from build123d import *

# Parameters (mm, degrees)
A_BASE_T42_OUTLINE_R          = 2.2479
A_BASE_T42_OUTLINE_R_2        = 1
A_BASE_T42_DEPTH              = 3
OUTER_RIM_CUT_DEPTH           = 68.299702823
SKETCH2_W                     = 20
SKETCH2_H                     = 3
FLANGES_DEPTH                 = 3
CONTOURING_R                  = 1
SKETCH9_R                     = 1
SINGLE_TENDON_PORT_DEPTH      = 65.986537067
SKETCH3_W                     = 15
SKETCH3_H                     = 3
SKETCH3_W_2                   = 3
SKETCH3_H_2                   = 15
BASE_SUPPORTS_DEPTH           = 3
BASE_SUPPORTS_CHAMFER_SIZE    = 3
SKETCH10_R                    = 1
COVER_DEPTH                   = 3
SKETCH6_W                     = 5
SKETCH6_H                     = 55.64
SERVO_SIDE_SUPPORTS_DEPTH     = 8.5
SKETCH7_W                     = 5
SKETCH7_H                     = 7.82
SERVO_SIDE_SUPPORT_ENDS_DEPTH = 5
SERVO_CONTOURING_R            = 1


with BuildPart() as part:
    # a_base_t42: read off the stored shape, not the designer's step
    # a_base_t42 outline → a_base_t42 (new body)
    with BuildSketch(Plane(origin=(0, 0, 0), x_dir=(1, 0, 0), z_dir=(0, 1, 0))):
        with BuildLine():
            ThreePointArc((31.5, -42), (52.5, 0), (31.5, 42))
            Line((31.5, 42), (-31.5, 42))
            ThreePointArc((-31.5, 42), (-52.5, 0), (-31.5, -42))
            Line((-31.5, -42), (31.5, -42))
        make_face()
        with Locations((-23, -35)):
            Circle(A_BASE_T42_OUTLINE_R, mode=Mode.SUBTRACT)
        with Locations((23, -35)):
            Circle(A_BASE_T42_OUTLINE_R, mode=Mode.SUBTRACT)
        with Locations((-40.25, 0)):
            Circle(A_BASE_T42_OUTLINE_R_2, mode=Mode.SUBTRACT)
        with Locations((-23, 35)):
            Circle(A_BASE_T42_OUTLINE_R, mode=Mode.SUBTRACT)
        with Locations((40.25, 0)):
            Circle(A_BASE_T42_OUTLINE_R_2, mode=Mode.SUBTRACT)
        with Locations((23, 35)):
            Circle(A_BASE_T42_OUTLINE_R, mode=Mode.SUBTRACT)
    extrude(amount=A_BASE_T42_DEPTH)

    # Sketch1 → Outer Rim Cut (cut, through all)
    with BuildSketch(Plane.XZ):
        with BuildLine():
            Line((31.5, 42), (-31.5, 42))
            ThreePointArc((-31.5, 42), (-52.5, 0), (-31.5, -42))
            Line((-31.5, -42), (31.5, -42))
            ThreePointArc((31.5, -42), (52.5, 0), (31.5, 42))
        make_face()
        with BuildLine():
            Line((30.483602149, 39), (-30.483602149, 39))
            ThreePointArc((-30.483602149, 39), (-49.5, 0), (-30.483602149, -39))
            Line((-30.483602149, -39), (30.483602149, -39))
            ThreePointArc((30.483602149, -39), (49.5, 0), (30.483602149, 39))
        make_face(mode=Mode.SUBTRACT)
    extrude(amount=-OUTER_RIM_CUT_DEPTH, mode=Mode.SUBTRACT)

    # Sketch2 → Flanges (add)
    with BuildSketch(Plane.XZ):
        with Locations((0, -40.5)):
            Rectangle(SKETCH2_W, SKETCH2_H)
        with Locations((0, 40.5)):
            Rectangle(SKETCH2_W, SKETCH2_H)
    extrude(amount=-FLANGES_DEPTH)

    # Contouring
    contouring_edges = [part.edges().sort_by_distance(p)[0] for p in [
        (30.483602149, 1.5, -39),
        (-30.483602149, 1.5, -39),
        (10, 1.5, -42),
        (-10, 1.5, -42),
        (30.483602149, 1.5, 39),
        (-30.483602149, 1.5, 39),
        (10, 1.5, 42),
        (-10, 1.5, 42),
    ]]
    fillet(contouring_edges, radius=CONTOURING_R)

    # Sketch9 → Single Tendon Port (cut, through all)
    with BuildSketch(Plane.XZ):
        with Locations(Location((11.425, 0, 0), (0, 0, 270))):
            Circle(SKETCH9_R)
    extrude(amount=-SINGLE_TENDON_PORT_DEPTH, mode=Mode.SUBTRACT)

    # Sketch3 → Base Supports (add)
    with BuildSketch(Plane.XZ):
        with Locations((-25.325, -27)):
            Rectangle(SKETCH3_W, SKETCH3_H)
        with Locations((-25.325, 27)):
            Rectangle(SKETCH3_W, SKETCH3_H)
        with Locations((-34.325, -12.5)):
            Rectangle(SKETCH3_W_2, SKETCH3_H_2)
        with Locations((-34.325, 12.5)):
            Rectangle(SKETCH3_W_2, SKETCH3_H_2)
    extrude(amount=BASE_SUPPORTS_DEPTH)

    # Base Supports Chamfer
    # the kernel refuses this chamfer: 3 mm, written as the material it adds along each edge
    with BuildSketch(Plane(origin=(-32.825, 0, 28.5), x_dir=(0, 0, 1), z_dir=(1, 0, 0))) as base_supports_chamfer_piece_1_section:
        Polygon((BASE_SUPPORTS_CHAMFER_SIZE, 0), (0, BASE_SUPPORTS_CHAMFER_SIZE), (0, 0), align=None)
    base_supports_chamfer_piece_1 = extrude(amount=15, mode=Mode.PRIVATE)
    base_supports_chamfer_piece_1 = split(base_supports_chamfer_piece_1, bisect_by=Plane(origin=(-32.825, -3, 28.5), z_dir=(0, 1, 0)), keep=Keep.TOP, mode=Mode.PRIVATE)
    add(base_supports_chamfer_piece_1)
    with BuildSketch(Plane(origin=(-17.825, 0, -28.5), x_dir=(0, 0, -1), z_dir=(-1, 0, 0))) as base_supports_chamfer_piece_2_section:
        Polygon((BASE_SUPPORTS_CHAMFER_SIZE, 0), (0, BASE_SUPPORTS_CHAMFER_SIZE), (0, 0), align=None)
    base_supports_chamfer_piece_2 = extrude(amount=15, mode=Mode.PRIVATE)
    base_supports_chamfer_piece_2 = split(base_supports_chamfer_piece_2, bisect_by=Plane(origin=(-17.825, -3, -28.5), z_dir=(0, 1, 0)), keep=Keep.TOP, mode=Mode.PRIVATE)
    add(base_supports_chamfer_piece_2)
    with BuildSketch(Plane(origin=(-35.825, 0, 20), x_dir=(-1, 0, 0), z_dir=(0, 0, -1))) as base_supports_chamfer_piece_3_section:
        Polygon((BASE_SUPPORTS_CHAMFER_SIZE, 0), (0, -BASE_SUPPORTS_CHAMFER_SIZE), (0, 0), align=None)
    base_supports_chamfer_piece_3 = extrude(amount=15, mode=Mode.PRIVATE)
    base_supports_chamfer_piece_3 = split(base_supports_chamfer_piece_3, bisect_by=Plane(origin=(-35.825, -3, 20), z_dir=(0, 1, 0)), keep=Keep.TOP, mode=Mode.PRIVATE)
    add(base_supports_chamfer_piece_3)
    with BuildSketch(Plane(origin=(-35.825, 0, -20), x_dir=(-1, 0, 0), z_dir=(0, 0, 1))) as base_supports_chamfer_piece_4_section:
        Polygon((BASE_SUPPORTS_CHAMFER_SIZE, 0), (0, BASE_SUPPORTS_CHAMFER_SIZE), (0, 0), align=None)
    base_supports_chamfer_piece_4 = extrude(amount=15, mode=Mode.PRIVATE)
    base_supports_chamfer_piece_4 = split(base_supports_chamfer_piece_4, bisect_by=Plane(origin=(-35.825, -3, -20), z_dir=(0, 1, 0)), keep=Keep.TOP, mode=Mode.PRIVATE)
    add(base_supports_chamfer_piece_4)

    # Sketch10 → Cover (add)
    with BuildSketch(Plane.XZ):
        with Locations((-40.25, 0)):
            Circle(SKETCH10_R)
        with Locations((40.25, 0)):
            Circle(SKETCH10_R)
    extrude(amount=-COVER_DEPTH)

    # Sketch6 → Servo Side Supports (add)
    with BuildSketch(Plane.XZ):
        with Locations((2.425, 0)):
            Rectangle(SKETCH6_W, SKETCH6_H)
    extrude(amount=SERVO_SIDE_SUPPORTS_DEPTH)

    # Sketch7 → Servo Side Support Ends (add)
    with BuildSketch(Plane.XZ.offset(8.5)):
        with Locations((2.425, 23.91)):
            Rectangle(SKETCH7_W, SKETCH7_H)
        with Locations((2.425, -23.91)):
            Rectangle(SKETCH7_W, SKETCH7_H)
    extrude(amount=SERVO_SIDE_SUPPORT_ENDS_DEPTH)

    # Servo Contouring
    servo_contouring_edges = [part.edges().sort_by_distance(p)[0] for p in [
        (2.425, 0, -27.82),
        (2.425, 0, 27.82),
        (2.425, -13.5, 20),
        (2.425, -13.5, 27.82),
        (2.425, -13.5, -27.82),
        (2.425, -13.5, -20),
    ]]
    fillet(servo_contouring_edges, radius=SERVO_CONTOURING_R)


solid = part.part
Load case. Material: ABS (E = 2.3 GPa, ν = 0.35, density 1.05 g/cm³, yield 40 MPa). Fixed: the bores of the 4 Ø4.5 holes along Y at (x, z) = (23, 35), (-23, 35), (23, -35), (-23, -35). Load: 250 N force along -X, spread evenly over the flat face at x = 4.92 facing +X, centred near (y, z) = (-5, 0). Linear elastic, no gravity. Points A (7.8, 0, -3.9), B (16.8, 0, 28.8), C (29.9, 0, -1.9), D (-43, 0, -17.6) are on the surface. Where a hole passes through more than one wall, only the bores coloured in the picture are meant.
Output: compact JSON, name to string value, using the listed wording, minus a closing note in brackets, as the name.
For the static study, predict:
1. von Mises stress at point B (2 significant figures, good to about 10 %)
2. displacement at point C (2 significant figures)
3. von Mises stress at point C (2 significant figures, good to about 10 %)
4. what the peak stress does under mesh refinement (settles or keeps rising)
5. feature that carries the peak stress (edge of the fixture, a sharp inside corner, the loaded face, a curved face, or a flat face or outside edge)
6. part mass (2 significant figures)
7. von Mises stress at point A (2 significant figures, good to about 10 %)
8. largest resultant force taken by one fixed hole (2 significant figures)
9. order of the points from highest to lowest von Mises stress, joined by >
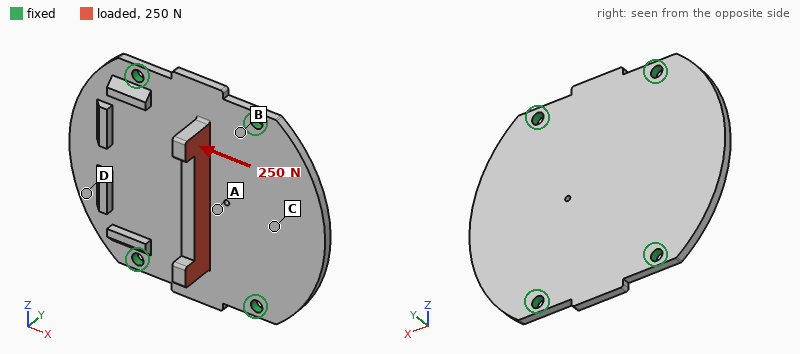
{"von Mises stress at point B": "2.4 MPa", "displacement at point C": "0.15 mm", "von Mises stress at point C": "1.3 MPa", "what the peak stress does under mesh refinement": "keeps rising", "feature that carries the peak stress": "a sharp inside corner", "part mass": "25 g", "von Mises stress at point A": "4.9 MPa", "largest resultant force taken by one fixed hole": "70 N", "order of the points from highest to lowest von Mises stress, joined by >": "A > B > C > D"}
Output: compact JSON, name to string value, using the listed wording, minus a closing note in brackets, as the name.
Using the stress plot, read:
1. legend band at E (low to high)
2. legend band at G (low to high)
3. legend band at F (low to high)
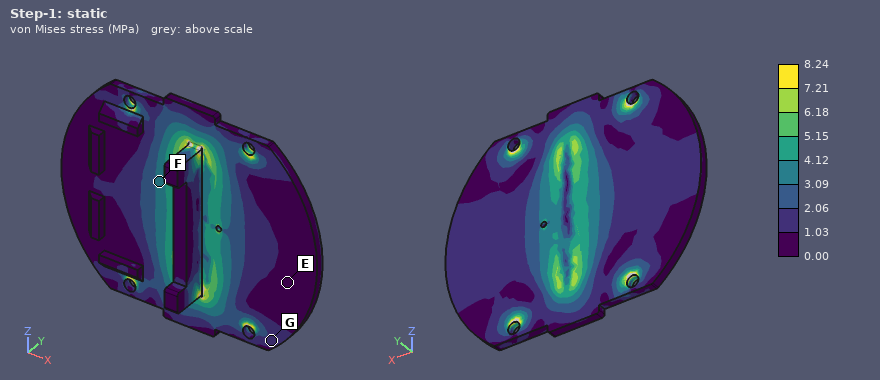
{"legend band at E": "0.00 to 1.03 MPa", "legend band at G": "1.03 to 2.06 MPa", "legend band at F": "3.09 to 4.12 MPa"}
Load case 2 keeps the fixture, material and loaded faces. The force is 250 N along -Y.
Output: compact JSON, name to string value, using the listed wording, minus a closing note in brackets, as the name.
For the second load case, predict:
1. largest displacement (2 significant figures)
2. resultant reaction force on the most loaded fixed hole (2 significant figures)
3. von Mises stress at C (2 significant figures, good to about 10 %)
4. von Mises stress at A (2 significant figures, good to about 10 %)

{"largest displacement": "0.67 mm", "resultant reaction force on the most loaded fixed hole": "82 N", "von Mises stress at C": "3.1 MPa", "von Mises stress at A": "8.2 MPa"}
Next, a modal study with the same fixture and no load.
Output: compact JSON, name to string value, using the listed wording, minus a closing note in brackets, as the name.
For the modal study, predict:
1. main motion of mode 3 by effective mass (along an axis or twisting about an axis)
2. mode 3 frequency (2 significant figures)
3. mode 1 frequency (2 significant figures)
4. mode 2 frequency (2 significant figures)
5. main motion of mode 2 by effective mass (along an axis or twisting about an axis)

{"main motion of mode 3 by effective mass": "along Y", "mode 3 frequency": "1100 Hz", "mode 1 frequency": "720 Hz", "mode 2 frequency": "780 Hz", "main motion of mode 2 by effective mass": "along Y"}
